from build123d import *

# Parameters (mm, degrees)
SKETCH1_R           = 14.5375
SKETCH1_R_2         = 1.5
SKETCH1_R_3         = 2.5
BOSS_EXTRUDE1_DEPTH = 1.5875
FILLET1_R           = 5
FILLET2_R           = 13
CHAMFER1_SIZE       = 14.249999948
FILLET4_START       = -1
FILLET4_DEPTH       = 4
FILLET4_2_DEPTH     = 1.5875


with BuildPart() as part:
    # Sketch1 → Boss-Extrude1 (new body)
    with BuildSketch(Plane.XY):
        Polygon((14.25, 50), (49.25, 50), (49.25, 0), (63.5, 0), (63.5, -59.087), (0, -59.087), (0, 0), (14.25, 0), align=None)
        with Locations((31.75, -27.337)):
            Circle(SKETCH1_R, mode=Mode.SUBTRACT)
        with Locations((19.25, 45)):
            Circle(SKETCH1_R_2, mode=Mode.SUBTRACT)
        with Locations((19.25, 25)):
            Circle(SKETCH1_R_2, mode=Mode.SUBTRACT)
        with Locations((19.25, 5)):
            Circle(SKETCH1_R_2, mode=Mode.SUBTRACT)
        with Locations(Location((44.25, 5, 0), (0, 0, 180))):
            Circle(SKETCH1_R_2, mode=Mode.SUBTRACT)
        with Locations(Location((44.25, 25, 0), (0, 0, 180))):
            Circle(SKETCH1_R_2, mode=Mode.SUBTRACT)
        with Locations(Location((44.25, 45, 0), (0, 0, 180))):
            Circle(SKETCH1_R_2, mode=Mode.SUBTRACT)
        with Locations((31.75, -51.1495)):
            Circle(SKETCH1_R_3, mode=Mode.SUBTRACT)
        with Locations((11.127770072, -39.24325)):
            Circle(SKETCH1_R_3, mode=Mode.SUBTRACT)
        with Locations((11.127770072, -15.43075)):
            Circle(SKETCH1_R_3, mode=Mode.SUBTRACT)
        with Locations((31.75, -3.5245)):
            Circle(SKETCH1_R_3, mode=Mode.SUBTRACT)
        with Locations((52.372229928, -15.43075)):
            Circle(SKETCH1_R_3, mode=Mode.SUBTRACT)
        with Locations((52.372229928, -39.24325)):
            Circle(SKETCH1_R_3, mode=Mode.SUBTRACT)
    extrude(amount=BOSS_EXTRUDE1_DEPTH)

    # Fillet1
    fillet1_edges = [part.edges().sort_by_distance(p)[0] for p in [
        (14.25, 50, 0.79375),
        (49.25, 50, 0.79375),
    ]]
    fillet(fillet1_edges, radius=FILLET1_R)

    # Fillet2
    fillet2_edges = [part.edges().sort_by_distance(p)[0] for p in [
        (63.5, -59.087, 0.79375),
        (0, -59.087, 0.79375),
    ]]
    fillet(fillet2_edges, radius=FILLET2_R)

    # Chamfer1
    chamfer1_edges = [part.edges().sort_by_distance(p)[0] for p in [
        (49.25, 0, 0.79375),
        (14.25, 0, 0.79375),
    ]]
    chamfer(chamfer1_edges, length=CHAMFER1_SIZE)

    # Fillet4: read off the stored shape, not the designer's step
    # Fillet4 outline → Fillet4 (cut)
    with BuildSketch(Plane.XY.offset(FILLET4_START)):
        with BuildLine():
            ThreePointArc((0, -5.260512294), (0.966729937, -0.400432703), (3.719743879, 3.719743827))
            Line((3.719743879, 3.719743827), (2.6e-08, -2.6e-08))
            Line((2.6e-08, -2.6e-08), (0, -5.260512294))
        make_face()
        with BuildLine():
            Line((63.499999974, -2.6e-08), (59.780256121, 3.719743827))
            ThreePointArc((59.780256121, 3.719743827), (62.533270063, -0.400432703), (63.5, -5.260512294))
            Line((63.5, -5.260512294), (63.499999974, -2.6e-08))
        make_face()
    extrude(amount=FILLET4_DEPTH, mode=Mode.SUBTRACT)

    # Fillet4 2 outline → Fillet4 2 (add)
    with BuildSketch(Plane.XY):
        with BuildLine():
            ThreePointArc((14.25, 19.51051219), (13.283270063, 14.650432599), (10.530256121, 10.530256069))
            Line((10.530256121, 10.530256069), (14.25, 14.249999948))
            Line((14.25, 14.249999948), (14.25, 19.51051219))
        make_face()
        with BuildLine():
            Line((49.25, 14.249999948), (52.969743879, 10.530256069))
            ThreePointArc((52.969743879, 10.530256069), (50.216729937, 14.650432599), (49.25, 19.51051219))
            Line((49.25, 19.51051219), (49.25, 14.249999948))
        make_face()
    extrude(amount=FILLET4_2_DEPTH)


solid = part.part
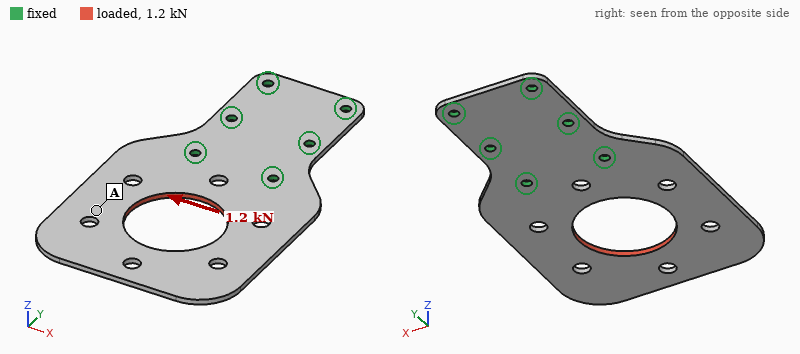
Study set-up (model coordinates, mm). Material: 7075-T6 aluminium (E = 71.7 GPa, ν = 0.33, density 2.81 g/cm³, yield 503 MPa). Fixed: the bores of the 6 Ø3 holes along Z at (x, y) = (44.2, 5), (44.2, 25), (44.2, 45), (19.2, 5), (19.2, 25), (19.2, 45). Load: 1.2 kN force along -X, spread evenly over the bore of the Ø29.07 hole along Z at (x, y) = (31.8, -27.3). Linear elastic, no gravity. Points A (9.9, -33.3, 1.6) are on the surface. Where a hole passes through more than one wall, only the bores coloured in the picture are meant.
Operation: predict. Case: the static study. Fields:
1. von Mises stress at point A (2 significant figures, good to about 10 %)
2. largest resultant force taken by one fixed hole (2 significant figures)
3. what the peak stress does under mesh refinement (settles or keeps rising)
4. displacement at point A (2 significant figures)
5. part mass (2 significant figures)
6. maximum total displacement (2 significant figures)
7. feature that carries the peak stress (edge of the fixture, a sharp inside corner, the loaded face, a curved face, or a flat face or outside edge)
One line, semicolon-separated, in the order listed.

17 MPa; 1.2 kN; keeps rising; 0.095 mm; 21 g; 0.14 mm; edge of the fixture
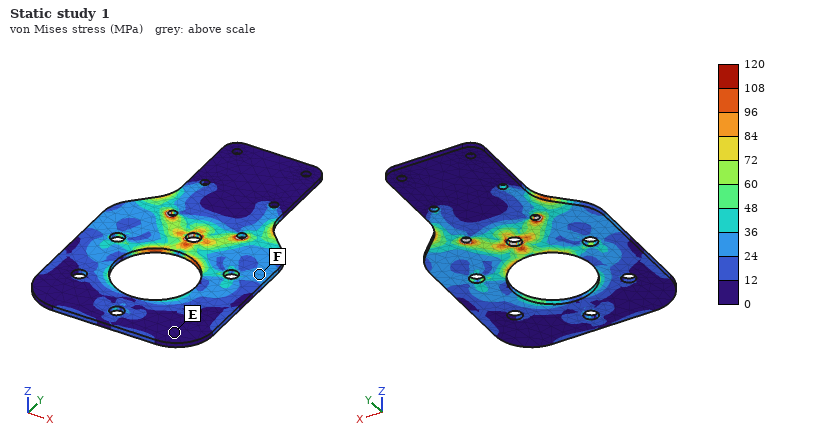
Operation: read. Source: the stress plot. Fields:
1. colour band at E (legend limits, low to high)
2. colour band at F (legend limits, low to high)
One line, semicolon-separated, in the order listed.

0 to 12 MPa; 24 to 36 MPa
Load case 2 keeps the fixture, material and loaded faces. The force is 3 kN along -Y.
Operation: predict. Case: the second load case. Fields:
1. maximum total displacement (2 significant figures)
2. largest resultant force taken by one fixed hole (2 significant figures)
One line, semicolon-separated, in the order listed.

55 µm; 1.2 kN
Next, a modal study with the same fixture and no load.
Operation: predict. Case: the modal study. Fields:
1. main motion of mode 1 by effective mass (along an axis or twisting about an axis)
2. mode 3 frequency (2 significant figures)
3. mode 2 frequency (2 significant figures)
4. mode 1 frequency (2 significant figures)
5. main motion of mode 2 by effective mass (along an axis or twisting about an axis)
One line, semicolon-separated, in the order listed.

along Z; 1600 Hz; 660 Hz; 290 Hz; twisting about Y
